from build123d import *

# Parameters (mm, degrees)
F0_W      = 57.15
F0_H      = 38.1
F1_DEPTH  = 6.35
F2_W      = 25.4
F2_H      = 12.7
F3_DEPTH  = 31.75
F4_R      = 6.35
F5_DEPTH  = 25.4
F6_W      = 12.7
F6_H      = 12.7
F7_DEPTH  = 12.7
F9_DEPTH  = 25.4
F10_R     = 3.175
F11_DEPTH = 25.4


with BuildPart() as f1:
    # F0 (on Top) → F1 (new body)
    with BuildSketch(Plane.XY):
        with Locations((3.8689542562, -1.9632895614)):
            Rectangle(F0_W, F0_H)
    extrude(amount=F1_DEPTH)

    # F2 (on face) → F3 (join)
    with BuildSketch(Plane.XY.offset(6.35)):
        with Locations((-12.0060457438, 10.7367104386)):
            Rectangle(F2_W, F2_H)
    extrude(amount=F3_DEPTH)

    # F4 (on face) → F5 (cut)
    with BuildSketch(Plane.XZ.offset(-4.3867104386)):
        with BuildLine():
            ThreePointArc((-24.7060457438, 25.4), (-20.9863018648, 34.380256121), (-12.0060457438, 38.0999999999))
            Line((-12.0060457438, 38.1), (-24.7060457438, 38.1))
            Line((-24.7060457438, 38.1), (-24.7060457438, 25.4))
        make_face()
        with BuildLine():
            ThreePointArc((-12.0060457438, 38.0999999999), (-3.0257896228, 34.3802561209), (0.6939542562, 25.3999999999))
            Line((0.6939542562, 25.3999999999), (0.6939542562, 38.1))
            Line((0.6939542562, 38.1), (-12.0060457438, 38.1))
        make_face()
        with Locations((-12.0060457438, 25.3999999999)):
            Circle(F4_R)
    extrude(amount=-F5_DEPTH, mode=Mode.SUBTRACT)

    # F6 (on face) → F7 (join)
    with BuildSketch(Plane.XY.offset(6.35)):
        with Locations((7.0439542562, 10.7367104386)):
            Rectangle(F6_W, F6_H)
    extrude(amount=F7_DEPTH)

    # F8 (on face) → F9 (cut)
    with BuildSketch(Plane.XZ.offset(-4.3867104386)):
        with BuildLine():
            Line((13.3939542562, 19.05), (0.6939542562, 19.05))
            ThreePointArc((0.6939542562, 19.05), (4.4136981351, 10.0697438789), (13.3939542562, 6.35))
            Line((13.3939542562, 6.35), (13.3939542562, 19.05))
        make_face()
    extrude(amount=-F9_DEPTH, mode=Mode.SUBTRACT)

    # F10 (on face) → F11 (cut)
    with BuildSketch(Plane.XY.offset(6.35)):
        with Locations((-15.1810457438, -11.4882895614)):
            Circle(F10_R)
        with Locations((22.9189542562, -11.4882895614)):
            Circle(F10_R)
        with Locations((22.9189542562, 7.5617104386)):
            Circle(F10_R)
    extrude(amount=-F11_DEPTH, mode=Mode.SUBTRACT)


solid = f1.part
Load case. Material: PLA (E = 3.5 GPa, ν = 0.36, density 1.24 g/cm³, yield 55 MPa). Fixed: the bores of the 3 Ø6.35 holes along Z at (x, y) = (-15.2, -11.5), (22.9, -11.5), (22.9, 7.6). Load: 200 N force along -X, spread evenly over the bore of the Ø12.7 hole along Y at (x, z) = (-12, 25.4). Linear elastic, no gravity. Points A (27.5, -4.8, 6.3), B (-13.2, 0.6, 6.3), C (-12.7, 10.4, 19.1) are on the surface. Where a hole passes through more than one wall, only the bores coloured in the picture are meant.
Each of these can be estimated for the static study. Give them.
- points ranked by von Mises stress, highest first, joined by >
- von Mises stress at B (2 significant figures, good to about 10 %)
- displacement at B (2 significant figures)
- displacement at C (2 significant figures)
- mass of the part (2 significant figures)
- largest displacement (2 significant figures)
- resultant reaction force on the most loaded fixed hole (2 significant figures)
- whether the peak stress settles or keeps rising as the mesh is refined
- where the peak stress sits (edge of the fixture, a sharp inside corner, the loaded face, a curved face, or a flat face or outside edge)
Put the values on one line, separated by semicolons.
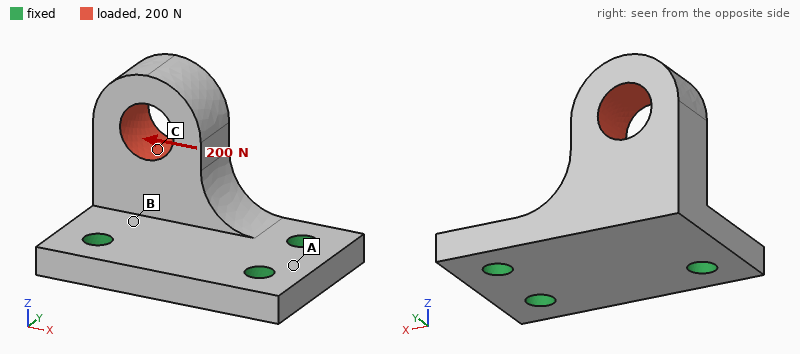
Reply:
B > C > A; 4.8 MPa; 0.047 mm; 0.15 mm; 27 g; 0.30 mm; 150 N; keeps rising; edge of the fixture
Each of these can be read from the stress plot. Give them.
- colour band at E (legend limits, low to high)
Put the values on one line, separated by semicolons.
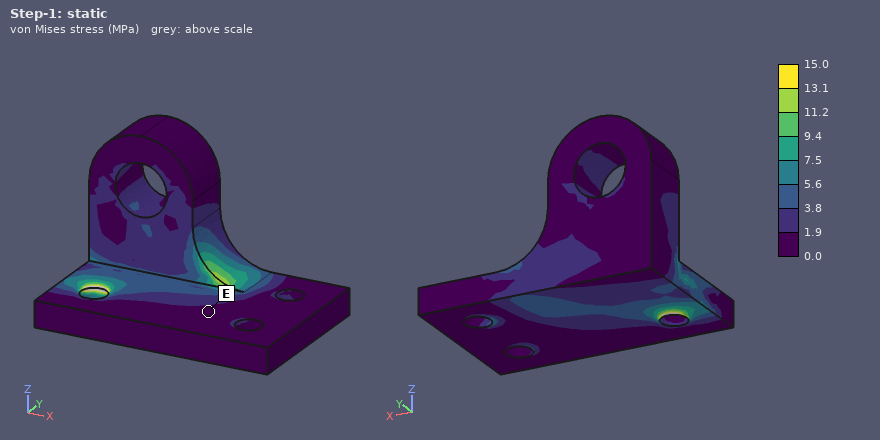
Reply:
0.0 to 1.9 MPa
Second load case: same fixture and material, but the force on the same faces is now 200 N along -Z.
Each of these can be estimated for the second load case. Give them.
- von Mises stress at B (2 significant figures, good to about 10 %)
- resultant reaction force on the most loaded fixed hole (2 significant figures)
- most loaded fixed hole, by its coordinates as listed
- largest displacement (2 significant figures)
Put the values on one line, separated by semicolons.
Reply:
4.6 MPa; 150 N; (-15.2, -11.5); 0.38 mm
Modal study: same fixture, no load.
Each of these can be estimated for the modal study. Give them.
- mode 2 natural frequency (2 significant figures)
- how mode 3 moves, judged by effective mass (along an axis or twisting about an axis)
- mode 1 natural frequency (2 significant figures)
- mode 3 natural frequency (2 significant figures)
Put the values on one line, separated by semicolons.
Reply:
2200 Hz; along Z; 1000 Hz; 3400 Hz
